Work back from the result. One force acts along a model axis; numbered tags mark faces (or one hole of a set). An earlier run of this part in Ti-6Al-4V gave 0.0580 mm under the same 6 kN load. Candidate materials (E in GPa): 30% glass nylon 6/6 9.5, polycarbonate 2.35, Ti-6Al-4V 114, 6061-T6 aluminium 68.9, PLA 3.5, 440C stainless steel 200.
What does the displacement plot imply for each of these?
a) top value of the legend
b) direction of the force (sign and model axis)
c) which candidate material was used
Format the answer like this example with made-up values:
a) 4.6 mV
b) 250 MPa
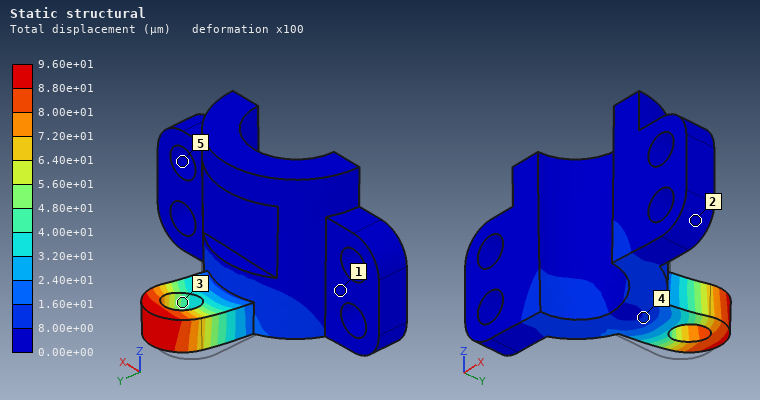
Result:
a) 9.60e+01 µm
b) +X
c) 6061-T6 aluminium
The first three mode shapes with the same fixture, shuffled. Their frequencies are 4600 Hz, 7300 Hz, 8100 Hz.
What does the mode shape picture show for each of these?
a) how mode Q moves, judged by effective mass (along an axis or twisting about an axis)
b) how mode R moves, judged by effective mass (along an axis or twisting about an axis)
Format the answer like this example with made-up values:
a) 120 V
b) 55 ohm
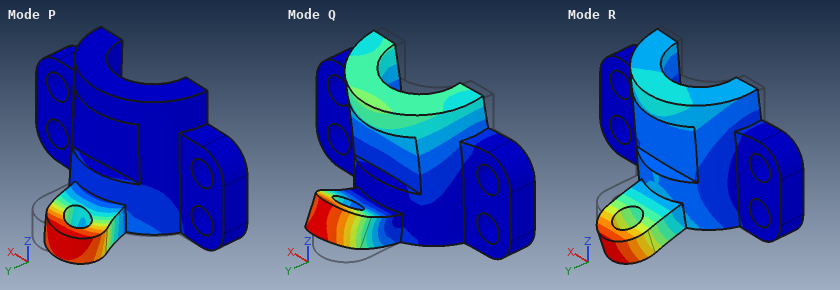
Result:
a) along Y
b) along Z
